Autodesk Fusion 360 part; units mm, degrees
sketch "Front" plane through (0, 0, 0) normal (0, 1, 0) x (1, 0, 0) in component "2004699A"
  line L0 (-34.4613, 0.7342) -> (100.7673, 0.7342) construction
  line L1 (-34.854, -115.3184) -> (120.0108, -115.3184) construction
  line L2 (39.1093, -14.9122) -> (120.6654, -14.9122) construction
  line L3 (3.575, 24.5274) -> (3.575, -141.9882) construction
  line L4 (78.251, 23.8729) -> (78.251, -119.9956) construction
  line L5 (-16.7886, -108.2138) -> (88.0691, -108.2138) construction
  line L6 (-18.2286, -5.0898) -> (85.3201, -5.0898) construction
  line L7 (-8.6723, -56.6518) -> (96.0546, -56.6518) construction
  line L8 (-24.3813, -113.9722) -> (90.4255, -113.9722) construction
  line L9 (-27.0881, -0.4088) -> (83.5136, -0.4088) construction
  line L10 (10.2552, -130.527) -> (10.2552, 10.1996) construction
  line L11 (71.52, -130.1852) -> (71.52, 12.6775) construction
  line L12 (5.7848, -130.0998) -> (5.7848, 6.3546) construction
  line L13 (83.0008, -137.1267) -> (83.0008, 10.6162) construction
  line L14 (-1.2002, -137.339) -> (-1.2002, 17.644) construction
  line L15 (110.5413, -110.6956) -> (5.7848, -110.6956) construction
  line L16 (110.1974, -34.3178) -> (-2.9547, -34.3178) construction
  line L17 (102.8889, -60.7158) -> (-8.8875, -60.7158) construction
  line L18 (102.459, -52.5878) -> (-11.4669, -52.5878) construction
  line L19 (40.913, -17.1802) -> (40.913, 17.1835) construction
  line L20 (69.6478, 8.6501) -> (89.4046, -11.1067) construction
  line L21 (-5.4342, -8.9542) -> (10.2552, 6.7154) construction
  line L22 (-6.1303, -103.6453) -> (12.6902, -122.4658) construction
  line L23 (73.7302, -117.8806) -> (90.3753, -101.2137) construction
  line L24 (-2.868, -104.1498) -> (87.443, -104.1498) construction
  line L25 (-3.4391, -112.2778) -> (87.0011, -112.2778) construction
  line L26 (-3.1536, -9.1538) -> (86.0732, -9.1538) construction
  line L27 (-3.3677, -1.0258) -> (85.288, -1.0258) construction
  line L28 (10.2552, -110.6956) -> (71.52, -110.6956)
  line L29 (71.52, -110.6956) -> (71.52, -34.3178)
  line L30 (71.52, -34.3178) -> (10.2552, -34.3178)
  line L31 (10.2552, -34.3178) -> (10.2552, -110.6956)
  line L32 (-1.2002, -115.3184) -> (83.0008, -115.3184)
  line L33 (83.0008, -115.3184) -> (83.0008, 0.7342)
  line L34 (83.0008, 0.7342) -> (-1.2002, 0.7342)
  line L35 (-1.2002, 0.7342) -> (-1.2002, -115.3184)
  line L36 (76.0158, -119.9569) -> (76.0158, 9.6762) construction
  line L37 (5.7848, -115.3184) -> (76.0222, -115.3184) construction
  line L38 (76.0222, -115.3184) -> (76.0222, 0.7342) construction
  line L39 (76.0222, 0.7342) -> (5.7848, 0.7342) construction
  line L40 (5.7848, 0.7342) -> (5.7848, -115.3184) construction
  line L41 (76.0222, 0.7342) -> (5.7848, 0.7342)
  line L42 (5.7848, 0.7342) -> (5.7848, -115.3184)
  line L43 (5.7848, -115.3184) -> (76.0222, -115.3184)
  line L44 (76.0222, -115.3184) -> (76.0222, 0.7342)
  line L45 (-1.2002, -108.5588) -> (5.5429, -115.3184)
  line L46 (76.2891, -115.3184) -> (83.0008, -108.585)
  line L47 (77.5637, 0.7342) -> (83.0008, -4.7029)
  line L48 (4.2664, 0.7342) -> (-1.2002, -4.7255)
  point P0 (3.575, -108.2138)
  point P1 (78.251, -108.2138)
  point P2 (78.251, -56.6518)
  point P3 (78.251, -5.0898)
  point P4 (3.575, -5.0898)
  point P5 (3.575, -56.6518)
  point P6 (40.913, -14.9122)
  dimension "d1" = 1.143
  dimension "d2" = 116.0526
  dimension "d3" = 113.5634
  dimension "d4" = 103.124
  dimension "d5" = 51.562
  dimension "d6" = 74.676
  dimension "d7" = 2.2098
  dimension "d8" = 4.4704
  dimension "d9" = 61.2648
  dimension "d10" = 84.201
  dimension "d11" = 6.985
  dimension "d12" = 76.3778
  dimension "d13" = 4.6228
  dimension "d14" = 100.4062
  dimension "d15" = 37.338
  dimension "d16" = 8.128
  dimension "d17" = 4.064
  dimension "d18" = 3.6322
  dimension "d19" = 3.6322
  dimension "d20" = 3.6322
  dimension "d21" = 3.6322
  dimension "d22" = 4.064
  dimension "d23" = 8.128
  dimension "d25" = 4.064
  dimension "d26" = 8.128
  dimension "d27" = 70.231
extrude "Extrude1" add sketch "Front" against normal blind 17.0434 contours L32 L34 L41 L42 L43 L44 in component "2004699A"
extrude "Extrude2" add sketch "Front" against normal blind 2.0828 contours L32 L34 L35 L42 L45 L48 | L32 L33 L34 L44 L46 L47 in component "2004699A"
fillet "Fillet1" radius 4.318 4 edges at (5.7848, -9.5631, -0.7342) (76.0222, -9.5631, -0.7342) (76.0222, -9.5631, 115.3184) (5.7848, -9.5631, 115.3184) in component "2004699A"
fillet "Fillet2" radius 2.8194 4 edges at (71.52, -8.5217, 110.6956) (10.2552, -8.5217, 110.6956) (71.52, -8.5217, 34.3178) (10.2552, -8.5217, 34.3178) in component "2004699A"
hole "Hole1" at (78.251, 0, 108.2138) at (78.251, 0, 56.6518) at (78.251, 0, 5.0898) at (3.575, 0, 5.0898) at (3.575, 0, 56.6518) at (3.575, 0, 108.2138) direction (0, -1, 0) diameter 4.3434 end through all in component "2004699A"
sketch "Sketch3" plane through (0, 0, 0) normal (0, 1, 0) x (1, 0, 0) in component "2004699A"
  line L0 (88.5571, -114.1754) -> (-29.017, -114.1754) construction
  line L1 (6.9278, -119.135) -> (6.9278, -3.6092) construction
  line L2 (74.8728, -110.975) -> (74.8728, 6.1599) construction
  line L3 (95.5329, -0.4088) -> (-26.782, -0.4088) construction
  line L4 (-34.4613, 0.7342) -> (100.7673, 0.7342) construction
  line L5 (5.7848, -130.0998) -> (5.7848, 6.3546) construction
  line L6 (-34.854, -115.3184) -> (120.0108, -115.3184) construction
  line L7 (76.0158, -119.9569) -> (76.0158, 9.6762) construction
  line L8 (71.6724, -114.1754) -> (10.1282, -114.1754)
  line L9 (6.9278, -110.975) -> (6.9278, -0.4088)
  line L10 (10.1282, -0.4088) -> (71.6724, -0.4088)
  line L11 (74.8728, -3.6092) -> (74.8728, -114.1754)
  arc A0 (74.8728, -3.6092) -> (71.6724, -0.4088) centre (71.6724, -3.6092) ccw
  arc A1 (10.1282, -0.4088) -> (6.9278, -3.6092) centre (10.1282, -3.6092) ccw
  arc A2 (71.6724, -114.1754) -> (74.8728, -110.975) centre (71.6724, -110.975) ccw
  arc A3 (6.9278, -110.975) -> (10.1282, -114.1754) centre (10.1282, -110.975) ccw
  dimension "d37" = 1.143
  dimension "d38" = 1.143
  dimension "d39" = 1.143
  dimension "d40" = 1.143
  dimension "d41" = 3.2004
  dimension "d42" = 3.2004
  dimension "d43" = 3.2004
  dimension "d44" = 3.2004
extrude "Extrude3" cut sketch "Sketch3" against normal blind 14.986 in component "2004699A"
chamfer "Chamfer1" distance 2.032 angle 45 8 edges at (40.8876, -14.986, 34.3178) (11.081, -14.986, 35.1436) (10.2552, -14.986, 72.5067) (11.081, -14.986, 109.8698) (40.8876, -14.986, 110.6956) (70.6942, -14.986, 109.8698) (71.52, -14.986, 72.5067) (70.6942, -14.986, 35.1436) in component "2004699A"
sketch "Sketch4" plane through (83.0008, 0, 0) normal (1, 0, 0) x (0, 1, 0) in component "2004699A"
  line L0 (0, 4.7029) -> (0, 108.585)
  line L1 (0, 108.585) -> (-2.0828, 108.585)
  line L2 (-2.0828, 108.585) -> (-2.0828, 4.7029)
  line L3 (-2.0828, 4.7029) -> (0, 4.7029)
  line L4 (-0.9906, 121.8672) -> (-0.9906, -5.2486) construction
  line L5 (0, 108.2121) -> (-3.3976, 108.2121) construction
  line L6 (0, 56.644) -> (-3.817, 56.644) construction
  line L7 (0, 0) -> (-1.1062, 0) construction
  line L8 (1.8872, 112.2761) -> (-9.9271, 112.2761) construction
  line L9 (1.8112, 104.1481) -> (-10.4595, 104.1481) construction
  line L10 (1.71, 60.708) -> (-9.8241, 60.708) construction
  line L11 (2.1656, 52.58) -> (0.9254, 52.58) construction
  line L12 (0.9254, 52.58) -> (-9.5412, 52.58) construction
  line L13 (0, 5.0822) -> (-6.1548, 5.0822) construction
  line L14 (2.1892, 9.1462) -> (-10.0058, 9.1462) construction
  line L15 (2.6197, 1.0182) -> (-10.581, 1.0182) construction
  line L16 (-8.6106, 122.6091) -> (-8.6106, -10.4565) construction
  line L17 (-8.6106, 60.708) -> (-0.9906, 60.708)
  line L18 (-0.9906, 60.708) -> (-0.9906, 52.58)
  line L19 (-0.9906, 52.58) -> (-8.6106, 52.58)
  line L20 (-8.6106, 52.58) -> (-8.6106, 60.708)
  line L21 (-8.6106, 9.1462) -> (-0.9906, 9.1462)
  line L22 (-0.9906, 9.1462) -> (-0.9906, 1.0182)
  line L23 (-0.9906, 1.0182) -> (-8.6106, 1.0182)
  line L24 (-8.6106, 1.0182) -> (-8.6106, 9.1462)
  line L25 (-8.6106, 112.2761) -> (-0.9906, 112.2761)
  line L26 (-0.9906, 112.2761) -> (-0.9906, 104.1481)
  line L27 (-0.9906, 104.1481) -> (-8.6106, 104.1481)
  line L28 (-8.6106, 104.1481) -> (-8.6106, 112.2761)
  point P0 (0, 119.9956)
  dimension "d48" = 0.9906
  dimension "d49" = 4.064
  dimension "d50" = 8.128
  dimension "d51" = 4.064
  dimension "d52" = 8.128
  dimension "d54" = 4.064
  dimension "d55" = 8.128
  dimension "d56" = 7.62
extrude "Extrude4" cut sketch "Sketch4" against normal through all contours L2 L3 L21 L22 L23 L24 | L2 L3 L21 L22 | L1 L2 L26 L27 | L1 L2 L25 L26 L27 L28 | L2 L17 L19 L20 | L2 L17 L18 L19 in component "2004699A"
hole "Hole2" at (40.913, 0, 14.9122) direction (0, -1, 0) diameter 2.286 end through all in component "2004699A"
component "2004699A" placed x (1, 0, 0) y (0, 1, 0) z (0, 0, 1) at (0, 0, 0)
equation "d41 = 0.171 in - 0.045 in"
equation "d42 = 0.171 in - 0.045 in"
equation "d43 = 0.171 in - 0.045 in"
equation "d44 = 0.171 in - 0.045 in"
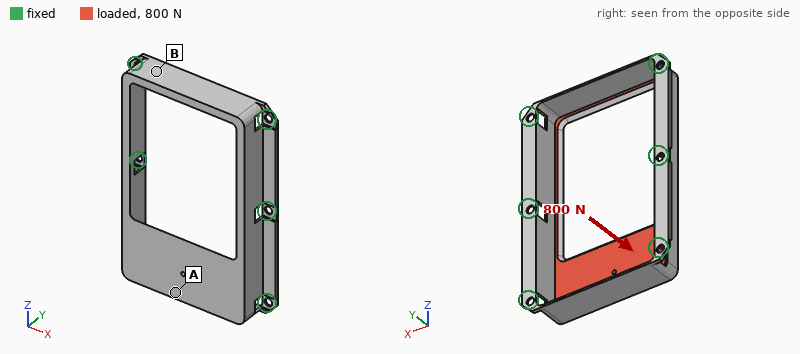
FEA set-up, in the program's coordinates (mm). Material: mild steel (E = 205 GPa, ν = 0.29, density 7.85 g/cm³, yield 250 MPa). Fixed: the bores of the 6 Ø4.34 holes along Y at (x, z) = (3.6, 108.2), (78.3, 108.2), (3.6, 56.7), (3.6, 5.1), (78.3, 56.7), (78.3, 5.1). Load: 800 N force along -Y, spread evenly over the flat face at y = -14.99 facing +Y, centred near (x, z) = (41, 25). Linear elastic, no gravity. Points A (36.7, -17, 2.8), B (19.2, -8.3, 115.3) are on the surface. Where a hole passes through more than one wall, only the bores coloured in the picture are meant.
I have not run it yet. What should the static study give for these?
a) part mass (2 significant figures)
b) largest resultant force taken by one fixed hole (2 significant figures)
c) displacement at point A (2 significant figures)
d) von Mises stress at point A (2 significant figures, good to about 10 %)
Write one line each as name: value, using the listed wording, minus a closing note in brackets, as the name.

part mass: 120 g
largest resultant force taken by one fixed hole: 330 N
displacement at point A: 0.034 mm
von Mises stress at point A: 28 MPa
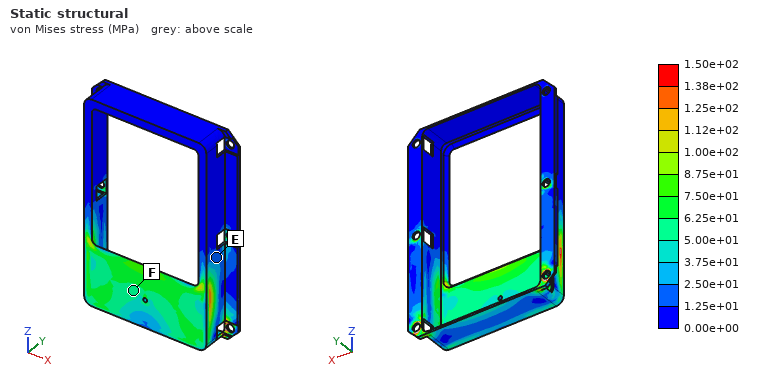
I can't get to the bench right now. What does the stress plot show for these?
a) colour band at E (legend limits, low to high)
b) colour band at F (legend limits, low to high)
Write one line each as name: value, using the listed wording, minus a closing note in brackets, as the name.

colour band at E: 1.25e+01 to 2.50e+01 MPa
colour band at F: 5.00e+01 to 6.25e+01 MPa
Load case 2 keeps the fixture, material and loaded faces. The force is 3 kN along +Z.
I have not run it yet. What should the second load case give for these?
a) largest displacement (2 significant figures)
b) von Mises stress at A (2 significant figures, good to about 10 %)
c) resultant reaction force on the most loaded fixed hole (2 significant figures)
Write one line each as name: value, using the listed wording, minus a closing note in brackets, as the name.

largest displacement: 61 µm
von Mises stress at A: 36 MPa
resultant reaction force on the most loaded fixed hole: 730 N
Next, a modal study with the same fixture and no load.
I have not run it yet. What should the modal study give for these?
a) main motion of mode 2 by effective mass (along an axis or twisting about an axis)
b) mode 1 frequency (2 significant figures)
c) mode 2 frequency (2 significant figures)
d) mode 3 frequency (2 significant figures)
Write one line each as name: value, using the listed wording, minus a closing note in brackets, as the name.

main motion of mode 2 by effective mass: along Y
mode 1 frequency: 2000 Hz
mode 2 frequency: 2100 Hz
mode 3 frequency: 3200 Hz
